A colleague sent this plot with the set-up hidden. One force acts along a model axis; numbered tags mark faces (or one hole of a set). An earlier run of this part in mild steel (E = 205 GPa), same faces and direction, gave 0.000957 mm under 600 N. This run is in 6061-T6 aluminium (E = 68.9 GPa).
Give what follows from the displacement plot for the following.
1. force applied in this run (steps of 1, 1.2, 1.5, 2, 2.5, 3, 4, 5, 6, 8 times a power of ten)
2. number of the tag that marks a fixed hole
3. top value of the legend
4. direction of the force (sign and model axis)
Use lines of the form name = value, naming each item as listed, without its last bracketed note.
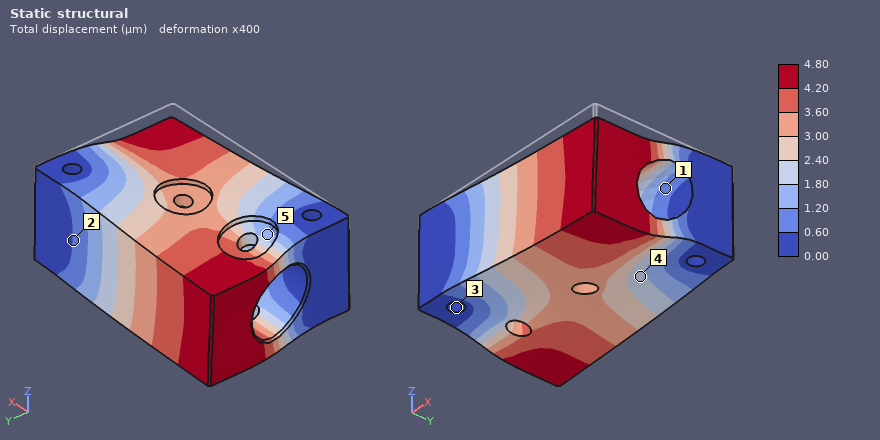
force applied in this run = 1 kN
number of the tag that marks a fixed hole = 3
top value of the legend = 4.80 µm
direction of the force = -Z
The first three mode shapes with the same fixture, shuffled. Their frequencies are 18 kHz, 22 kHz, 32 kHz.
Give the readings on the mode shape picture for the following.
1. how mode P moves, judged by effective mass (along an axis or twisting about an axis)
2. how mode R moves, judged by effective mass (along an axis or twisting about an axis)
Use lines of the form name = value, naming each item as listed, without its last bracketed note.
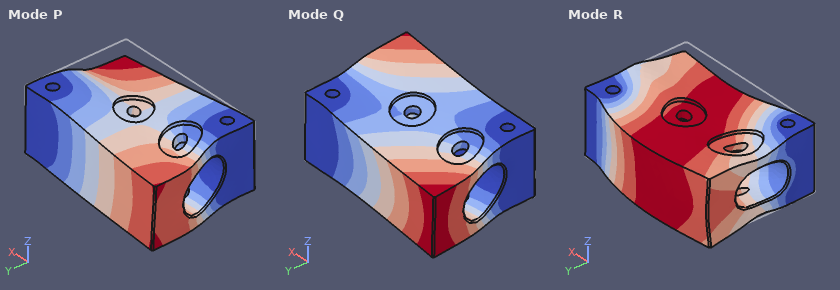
how mode P moves, judged by effective mass = along Z
how mode R moves, judged by effective mass = along Y
